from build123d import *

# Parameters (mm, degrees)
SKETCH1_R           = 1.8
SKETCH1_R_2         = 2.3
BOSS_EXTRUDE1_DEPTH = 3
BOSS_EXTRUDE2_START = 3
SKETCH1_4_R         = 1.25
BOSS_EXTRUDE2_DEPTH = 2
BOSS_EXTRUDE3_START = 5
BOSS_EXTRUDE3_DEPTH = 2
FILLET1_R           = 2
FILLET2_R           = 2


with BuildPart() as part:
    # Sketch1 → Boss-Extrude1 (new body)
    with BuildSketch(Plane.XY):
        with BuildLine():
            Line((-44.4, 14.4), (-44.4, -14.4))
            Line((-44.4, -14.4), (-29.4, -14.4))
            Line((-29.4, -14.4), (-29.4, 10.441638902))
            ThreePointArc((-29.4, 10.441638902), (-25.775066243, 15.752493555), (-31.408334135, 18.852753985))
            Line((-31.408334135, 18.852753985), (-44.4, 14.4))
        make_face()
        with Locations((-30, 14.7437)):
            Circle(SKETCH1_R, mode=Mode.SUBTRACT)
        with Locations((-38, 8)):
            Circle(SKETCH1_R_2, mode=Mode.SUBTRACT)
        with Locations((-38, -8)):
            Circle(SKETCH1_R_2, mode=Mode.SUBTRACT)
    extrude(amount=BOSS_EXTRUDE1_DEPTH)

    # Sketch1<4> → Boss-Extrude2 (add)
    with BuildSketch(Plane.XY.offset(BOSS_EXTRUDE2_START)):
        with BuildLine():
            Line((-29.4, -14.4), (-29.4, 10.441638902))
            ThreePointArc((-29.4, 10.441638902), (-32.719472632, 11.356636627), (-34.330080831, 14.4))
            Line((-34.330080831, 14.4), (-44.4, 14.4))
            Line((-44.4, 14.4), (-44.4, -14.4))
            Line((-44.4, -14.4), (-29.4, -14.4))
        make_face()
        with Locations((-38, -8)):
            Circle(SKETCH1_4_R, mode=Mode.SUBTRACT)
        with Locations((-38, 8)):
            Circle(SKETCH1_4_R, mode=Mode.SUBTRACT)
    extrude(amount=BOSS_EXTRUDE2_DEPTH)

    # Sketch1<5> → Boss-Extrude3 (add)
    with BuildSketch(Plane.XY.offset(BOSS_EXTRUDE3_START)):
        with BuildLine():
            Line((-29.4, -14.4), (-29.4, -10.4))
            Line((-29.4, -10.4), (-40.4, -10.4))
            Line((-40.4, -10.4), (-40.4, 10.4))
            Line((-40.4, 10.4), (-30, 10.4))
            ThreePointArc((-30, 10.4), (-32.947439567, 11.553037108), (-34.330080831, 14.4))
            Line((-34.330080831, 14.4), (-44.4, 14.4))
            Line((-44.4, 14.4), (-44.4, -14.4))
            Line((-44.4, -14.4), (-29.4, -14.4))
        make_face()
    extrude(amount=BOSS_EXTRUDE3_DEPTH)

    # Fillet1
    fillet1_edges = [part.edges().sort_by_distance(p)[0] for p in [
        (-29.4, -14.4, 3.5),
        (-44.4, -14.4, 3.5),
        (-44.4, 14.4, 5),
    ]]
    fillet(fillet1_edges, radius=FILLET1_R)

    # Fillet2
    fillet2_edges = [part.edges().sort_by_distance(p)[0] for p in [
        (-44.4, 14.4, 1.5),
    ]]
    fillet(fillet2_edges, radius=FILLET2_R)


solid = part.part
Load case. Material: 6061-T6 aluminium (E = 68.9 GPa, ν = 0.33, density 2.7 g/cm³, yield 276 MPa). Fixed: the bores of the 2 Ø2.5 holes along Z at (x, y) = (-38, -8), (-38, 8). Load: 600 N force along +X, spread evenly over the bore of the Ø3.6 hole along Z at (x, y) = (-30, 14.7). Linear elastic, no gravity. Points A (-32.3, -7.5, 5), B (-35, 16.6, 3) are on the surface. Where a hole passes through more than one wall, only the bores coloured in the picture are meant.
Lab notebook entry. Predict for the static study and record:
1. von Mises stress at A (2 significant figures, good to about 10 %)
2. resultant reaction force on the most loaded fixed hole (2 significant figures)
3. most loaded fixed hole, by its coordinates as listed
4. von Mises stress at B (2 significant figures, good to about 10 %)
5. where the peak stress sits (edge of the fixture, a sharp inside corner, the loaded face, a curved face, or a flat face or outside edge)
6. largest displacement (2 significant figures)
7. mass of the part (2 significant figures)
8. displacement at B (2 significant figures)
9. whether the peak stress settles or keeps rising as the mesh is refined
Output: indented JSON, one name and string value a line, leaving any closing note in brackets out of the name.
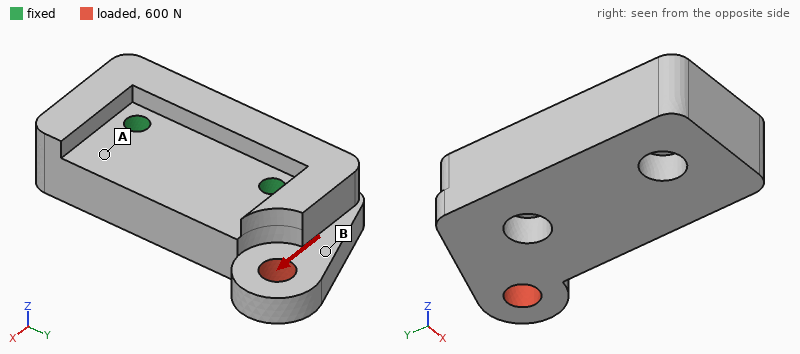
{
  "von Mises stress at A": "11 MPa",
  "resultant reaction force on the most loaded fixed hole": "810 N",
  "most loaded fixed hole, by its coordinates as listed": "(-38, 8)",
  "von Mises stress at B": "33 MPa",
  "where the peak stress sits": "edge of the fixture",
  "largest displacement": "33 µm",
  "mass of the part": "6.8 g",
  "displacement at B": "14 µm",
  "whether the peak stress settles or keeps rising as the mesh is refined": "keeps rising"
}
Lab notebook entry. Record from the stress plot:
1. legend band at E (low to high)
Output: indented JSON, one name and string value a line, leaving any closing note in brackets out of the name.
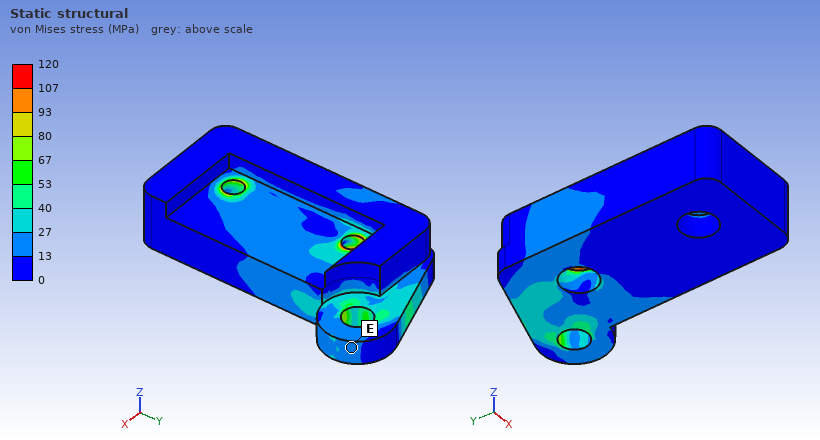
{
  "legend band at E": "13 to 27 MPa"
}
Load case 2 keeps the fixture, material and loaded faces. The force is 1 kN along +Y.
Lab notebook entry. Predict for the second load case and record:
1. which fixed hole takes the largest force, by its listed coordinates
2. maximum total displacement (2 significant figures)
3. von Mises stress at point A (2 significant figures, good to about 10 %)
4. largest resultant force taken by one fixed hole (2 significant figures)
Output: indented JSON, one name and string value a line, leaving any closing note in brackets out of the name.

{
  "which fixed hole takes the largest force, by its listed coordinates": "(-38, 8)",
  "maximum total displacement": "33 µm",
  "von Mises stress at point A": "13 MPa",
  "largest resultant force taken by one fixed hole": "740 N"
}
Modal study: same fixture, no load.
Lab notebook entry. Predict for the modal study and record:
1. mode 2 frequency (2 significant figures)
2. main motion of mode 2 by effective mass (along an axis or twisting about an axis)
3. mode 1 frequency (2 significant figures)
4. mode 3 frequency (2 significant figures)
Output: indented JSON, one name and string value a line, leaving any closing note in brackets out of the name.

{
  "mode 2 frequency": "22 kHz",
  "main motion of mode 2 by effective mass": "twisting about X",
  "mode 1 frequency": "13 kHz",
  "mode 3 frequency": "30 kHz"
}
